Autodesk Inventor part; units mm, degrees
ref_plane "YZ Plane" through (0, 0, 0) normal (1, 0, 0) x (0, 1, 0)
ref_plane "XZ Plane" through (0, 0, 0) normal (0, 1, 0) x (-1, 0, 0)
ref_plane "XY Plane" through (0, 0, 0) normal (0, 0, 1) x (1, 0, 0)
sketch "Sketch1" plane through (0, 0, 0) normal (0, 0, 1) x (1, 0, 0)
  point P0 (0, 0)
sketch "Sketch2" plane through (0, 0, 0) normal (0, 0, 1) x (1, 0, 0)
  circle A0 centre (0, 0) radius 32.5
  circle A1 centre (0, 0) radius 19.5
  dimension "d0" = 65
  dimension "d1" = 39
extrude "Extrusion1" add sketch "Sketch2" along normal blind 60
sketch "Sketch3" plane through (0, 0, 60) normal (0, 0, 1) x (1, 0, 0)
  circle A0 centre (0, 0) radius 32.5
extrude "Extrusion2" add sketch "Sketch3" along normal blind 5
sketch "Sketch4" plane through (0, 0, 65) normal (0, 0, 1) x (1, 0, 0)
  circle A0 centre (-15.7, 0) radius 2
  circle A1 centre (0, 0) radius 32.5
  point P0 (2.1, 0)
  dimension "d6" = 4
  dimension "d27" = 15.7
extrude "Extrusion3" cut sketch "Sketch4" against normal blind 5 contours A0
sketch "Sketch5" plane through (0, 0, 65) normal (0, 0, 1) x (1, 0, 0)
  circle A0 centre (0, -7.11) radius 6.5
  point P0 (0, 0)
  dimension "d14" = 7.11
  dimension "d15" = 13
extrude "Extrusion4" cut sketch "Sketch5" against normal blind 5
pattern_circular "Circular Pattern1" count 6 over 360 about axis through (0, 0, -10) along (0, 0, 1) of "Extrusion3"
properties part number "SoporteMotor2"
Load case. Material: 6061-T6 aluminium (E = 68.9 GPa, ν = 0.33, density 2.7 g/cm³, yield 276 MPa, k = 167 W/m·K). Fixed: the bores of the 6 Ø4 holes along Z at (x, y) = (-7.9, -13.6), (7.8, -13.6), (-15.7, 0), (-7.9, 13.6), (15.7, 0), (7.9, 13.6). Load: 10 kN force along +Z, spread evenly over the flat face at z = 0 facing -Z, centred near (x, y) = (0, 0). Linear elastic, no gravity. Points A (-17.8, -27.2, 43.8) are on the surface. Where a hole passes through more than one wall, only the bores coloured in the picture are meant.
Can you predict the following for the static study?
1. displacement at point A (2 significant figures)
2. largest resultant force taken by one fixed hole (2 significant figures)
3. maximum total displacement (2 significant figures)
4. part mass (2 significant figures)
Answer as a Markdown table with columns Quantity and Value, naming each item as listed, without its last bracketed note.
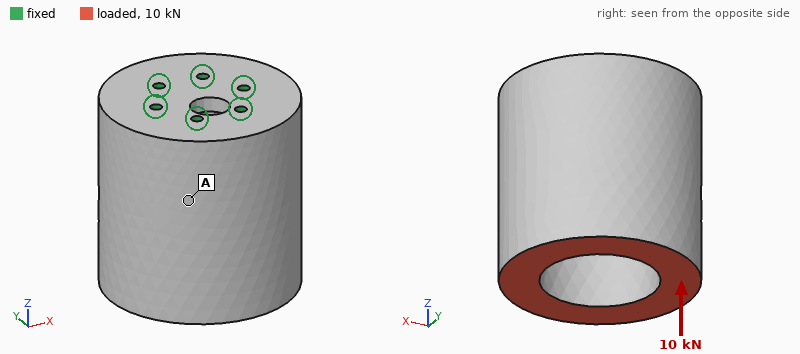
| Quantity | Value |
|---|---|
| displacement at point A | 10 µm |
| largest resultant force taken by one fixed hole | 1.7 kN |
| maximum total displacement | 13 µm |
| part mass | 390 g |
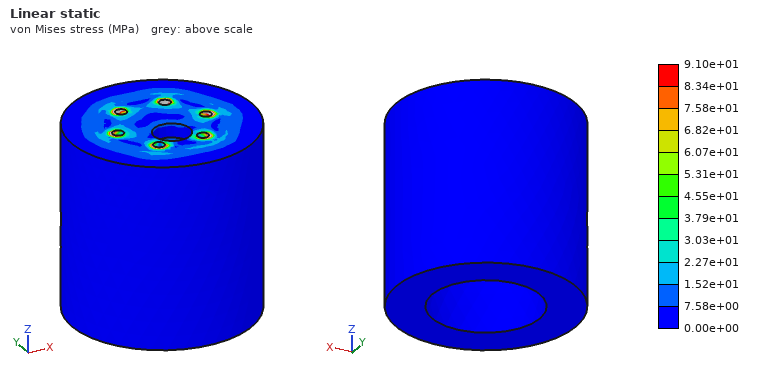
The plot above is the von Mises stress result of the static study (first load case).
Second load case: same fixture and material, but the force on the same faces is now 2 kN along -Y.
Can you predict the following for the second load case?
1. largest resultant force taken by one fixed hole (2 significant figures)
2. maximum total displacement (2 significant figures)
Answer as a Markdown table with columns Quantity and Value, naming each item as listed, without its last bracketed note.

| Quantity | Value |
|---|---|
| largest resultant force taken by one fixed hole | 1.9 kN |
| maximum total displacement | 57 µm |
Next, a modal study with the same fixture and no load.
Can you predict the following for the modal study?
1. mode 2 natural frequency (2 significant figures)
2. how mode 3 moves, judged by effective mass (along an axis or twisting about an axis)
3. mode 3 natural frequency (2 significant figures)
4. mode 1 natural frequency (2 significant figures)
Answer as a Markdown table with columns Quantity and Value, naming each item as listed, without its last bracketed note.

| Quantity | Value |
|---|---|
| mode 2 natural frequency | 2600 Hz |
| how mode 3 moves, judged by effective mass | twisting about Z |
| mode 3 natural frequency | 7400 Hz |
| mode 1 natural frequency | 2600 Hz |
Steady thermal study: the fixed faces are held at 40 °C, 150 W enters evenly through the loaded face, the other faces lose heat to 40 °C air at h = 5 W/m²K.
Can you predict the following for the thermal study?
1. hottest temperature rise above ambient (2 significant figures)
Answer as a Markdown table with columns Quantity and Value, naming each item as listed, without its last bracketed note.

| Quantity | Value |
|---|---|
| hottest temperature rise above ambient | 37 K |
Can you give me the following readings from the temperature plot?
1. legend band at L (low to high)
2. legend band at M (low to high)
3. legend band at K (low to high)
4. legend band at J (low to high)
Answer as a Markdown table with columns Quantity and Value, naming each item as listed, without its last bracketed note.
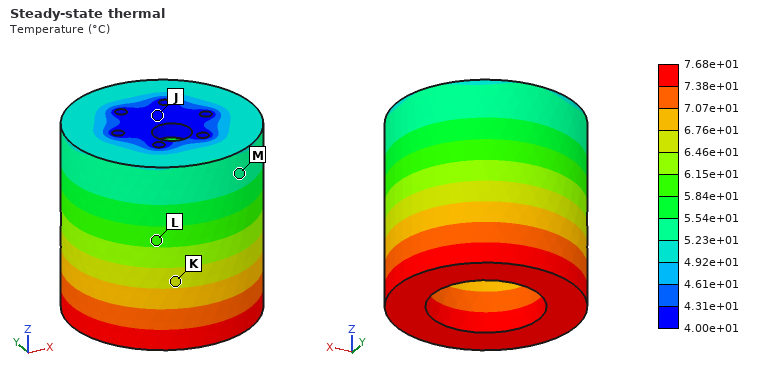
| Quantity | Value |
|---|---|
| legend band at L | 5.84e+01 to 6.15e+01 °C |
| legend band at M | 5.23e+01 to 5.54e+01 °C |
| legend band at K | 6.46e+01 to 6.76e+01 °C |
| legend band at J | 4.00e+01 to 4.31e+01 °C |
